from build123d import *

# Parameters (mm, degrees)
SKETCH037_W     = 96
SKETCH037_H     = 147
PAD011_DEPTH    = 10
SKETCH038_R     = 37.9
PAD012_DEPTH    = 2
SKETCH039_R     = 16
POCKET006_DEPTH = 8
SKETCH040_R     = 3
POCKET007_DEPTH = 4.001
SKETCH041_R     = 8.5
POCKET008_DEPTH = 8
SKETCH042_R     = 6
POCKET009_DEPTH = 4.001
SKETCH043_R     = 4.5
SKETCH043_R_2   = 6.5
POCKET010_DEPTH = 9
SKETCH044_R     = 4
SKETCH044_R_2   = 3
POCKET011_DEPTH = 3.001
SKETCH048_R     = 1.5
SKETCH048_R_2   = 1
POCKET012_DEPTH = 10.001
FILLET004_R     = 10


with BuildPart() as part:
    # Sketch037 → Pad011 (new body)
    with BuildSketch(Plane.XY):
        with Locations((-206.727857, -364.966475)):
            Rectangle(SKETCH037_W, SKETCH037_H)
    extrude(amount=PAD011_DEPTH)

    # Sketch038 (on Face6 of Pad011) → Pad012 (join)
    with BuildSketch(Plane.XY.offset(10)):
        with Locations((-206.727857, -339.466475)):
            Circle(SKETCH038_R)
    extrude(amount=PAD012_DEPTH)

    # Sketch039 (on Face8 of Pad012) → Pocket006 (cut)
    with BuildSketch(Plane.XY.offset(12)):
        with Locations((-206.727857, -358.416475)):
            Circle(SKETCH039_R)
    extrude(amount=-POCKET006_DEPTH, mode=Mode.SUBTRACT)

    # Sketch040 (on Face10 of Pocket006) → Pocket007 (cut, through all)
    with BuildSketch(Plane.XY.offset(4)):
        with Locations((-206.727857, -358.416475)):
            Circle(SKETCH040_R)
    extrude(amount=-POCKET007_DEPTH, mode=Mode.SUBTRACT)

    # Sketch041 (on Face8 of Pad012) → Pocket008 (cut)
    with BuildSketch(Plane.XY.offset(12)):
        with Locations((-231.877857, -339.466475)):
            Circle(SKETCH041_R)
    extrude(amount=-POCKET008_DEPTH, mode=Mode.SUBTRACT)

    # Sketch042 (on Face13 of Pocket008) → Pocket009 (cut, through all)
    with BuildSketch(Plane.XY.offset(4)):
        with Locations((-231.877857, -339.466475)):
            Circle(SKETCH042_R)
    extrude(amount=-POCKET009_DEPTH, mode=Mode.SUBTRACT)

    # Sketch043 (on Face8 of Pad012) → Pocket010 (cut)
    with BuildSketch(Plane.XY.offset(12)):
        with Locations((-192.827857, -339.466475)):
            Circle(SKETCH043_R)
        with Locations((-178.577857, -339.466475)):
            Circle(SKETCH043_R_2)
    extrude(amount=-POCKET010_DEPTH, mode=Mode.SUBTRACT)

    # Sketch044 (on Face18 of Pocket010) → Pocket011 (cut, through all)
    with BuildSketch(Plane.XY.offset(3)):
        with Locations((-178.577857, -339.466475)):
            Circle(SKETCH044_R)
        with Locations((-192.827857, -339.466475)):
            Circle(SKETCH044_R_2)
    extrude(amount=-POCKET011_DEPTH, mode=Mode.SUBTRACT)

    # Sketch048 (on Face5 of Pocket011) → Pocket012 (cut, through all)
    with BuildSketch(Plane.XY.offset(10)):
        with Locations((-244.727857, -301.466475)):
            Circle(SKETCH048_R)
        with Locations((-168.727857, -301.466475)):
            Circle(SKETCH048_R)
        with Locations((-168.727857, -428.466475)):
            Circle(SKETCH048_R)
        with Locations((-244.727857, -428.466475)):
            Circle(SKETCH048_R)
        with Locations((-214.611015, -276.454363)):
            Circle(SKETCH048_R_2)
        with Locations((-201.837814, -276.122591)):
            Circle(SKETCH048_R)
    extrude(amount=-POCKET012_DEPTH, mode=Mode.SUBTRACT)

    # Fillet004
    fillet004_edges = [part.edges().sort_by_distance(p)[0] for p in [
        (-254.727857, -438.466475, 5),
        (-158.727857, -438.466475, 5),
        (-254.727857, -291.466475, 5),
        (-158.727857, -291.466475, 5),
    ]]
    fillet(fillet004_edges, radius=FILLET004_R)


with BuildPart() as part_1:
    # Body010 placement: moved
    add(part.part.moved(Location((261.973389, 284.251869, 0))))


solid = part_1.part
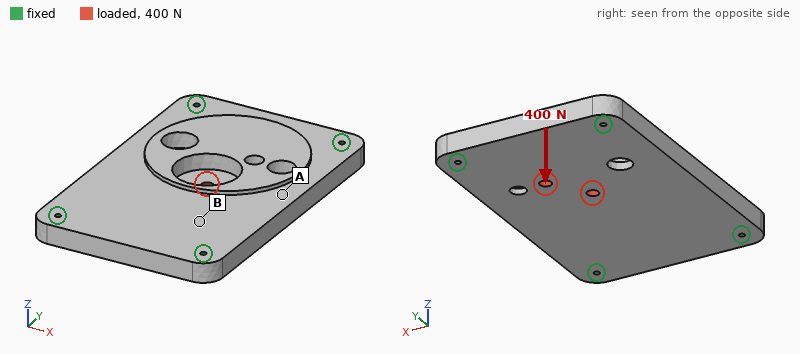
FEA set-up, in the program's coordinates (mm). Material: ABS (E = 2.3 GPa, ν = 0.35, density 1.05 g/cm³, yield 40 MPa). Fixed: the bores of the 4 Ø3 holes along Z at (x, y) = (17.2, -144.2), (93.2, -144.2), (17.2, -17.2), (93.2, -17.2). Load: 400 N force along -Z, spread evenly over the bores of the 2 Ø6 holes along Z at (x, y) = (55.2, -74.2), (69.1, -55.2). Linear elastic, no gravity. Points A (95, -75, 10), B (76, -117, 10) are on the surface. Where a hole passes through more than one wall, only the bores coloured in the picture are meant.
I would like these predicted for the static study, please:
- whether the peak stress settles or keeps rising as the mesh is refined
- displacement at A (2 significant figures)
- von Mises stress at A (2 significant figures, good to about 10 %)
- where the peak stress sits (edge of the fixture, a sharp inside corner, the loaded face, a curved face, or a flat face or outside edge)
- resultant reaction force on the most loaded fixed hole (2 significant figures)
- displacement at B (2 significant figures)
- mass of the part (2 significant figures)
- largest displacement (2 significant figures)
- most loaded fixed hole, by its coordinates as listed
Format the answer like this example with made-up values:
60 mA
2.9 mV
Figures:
keeps rising
0.33 mm
3.0 MPa
edge of the fixture
160 N
0.18 mm
150 g
0.57 mm
(93.2, -17.2)
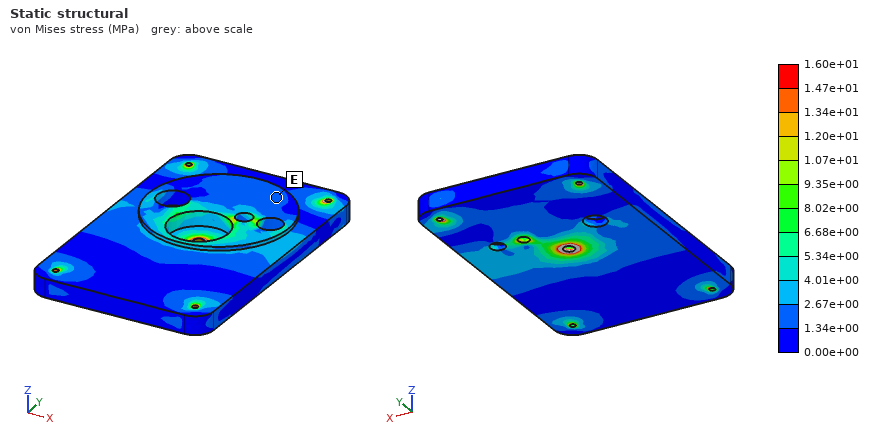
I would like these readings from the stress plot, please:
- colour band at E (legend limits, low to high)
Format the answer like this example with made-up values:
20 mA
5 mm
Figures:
1.34e+00 to 2.67e+00 MPa
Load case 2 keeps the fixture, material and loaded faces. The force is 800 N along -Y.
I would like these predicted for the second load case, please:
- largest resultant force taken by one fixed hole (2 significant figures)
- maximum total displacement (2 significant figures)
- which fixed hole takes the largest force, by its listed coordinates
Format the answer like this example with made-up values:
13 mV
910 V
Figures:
260 N
58 µm
(93.2, -17.2)
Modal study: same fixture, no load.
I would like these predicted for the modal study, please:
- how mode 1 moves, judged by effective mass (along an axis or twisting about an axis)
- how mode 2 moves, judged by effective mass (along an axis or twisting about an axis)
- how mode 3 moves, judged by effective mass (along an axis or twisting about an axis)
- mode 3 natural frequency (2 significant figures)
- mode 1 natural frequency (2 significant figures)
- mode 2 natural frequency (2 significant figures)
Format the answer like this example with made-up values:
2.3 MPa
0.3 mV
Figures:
along Z
twisting about Y
twisting about X
1700 Hz
690 Hz
1100 Hz
